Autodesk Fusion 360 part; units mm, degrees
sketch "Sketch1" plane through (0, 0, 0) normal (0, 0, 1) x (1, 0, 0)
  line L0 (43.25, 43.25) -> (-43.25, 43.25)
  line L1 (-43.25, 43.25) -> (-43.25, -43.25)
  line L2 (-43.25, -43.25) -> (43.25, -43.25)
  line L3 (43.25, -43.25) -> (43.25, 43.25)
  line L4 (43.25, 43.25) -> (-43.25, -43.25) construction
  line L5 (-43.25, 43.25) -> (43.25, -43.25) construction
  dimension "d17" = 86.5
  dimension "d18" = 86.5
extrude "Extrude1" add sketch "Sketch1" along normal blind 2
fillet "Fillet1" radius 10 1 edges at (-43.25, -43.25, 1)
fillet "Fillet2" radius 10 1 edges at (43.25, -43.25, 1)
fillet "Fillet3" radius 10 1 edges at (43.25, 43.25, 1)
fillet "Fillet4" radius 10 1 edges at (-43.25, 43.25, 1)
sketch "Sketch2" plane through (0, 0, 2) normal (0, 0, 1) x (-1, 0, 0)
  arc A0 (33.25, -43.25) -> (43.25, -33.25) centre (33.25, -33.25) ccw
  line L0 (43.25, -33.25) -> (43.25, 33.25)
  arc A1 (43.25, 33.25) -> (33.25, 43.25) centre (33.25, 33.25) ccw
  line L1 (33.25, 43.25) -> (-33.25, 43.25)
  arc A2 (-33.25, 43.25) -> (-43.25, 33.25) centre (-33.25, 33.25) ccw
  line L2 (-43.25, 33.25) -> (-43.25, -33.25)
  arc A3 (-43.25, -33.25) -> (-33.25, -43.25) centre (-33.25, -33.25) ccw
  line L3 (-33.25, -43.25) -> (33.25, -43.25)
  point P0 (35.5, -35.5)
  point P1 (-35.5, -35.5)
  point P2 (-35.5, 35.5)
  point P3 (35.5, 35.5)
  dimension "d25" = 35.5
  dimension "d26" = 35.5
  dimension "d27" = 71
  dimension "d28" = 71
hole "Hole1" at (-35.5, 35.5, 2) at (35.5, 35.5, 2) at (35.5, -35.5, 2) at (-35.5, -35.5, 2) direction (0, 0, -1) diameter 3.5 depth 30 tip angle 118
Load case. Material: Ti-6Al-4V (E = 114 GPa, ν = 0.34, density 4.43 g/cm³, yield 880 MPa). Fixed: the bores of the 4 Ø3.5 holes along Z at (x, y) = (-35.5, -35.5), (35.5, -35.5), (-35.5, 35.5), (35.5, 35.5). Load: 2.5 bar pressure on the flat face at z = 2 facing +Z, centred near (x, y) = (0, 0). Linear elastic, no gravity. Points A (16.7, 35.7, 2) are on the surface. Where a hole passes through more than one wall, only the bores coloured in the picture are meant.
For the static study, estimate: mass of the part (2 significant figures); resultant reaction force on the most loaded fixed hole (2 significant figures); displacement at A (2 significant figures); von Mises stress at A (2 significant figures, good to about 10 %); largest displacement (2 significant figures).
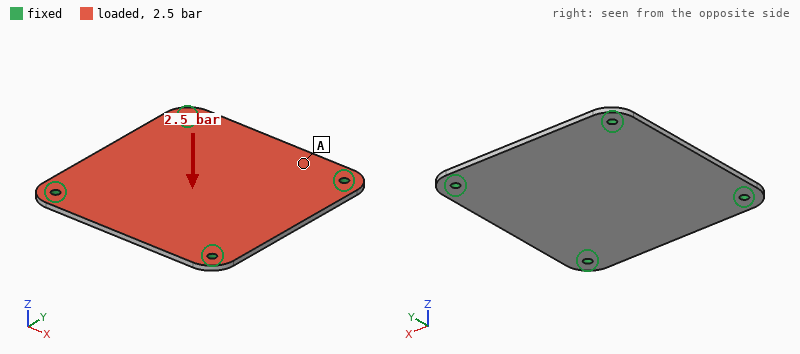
65 g
460 N
0.19 mm
48 MPa
0.55 mm
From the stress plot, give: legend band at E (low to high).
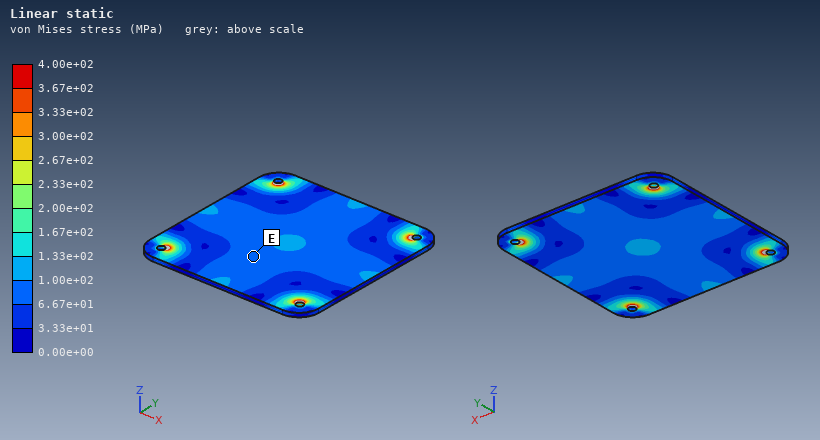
6.67e+01 to 1.00e+02 MPa
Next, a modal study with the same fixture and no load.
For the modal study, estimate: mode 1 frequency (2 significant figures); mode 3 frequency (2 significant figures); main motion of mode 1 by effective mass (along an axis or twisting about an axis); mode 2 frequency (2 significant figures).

1400 Hz
2300 Hz
along Z
2300 Hz
